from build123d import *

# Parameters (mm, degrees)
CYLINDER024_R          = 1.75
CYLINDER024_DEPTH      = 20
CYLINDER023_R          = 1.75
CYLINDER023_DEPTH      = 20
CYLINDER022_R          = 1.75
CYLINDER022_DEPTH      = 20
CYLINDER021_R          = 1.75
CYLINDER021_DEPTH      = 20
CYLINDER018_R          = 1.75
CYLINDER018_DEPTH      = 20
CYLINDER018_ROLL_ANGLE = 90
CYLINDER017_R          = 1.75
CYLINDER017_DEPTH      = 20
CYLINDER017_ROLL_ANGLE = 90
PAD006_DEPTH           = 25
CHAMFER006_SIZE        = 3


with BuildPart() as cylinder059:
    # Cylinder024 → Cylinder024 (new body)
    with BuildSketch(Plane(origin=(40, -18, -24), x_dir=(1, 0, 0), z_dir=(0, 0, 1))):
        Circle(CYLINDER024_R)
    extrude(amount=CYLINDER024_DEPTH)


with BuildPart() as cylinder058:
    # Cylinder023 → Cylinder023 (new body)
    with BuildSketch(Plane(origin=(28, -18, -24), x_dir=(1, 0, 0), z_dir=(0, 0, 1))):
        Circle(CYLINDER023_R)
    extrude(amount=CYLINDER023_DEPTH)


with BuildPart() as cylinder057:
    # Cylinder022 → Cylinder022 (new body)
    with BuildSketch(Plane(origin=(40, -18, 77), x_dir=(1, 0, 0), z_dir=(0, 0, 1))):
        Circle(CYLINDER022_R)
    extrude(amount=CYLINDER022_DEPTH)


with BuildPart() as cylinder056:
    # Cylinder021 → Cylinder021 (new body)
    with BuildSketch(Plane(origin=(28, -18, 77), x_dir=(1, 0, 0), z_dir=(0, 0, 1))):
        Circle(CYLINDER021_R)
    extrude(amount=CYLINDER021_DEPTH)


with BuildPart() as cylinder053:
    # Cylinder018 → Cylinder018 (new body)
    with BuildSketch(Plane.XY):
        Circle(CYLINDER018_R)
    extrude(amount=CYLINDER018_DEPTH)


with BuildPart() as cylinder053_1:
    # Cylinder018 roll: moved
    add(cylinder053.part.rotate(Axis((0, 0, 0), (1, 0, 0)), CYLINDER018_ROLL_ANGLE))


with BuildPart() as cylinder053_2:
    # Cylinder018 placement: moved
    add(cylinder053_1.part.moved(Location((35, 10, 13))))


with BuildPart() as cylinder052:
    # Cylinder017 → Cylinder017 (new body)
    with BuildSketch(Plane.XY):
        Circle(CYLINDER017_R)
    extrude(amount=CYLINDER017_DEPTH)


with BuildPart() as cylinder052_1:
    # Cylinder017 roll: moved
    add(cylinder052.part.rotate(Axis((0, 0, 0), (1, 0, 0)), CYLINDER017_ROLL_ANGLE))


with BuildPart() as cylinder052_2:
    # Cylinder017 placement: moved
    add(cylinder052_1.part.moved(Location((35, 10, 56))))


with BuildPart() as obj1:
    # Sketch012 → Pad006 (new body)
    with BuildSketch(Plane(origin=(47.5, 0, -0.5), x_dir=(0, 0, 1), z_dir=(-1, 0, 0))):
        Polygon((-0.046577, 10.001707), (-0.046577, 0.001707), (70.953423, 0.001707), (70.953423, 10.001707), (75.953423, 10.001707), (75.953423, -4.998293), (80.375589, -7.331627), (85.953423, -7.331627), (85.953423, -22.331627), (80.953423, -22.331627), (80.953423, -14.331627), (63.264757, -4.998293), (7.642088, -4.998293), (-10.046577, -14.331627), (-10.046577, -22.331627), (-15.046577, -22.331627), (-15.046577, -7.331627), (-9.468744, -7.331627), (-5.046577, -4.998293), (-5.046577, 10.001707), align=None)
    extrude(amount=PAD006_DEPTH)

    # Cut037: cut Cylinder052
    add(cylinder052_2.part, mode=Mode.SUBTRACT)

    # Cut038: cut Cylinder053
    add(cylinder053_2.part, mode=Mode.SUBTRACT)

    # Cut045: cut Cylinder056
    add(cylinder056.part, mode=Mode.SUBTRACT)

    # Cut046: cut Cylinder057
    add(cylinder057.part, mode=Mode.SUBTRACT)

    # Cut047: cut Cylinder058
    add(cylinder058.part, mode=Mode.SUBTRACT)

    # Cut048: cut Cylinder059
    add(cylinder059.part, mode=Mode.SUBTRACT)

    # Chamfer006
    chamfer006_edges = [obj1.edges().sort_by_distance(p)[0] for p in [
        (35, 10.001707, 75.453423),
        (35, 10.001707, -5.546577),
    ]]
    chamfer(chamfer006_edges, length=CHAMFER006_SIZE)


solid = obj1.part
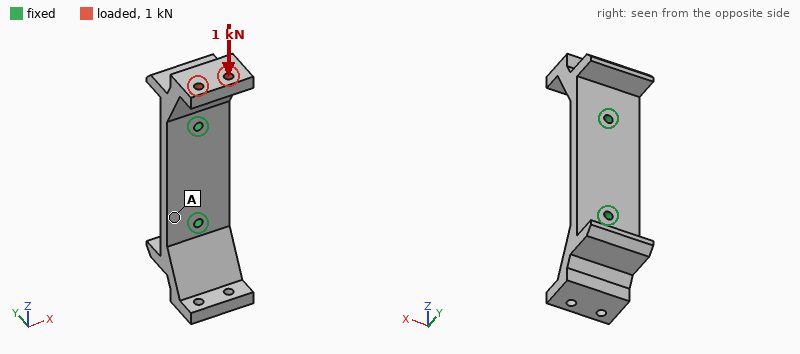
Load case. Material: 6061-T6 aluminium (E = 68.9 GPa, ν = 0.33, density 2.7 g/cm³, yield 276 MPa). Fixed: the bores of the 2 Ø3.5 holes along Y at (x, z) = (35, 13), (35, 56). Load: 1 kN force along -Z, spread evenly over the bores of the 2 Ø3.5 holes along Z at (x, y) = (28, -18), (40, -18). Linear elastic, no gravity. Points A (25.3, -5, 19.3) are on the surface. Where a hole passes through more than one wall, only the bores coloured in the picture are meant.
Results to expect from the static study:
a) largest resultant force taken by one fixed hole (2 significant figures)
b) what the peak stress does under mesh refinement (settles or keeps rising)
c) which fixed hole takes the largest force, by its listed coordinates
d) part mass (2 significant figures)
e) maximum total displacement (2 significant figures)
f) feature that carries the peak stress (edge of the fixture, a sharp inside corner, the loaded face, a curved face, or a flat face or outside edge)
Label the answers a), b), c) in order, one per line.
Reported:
a) 880 N
b) keeps rising
c) (35, 56)
d) 53 g
e) 0.38 mm
f) edge of the fixture
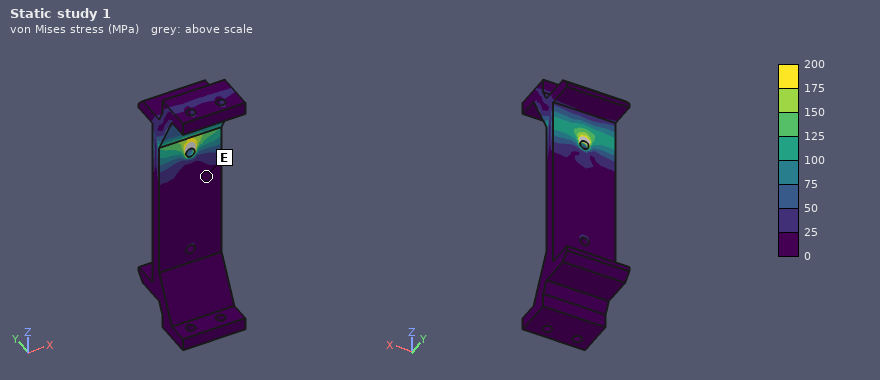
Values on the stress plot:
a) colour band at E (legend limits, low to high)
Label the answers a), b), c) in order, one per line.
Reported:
a) 0 to 25 MPa
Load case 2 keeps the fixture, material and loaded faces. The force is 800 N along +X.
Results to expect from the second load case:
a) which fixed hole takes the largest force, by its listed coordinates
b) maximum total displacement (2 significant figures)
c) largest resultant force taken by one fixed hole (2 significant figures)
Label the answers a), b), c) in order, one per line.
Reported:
a) (35, 56)
b) 0.16 mm
c) 1.2 kN
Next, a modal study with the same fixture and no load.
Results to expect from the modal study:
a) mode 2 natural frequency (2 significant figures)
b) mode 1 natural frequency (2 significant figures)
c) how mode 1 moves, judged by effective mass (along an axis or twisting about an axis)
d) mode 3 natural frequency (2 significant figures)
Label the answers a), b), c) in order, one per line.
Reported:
a) 2800 Hz
b) 2600 Hz
c) along Y
d) 4900 Hz
